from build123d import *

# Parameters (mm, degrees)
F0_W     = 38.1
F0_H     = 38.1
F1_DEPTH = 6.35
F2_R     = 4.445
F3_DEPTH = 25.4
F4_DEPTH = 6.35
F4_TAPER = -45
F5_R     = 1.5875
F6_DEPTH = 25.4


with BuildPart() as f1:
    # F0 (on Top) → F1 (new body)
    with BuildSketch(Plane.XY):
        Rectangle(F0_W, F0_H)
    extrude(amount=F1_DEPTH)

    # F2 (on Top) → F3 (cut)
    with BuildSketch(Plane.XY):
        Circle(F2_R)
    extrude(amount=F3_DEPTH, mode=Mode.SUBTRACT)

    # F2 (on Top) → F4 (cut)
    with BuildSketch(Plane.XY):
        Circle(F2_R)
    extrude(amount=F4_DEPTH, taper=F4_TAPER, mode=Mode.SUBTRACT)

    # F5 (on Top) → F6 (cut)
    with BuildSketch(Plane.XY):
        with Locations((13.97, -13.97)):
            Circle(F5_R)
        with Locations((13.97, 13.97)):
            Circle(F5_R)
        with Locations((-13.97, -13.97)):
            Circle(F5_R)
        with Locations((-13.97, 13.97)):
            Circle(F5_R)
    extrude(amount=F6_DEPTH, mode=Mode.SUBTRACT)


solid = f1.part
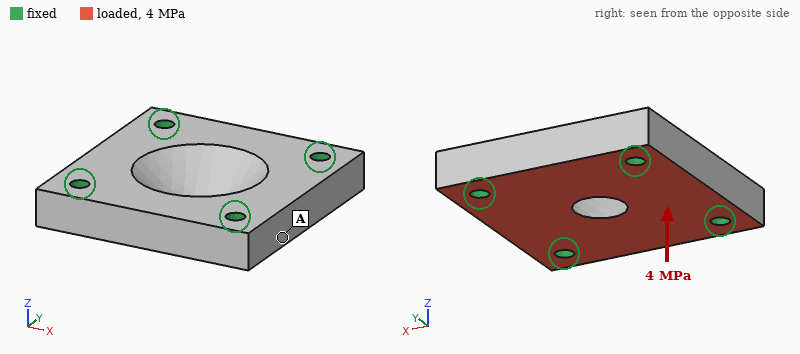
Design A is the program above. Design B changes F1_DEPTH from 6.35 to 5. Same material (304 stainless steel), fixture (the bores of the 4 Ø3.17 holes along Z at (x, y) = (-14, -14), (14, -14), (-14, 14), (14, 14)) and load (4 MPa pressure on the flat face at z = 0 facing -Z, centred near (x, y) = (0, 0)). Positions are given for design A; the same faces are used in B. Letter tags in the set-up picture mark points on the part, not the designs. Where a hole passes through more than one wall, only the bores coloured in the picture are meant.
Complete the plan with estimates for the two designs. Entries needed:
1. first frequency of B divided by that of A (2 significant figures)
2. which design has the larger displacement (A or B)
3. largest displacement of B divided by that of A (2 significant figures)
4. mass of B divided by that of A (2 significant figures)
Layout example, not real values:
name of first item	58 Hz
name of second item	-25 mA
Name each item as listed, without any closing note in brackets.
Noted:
first frequency of B divided by that of A	0.84
which design has the larger displacement	B
largest displacement of B divided by that of A	1.6
mass of B divided by that of A	0.81
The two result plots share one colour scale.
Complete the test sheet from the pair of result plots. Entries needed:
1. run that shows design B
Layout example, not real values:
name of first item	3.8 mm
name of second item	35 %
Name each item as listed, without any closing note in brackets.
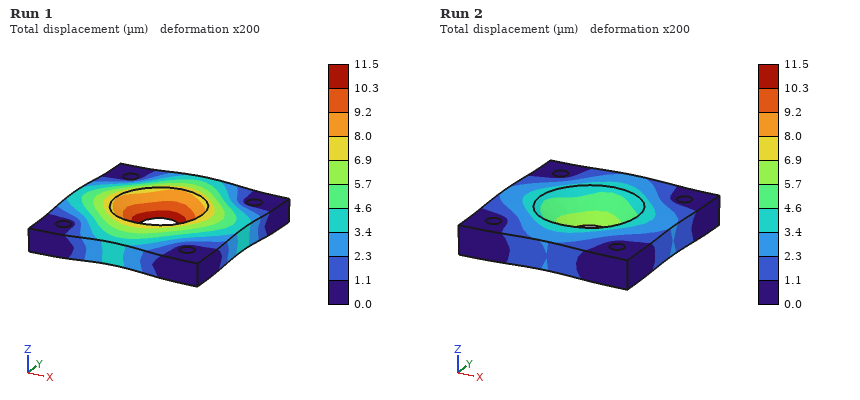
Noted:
run that shows design B	Run 1
